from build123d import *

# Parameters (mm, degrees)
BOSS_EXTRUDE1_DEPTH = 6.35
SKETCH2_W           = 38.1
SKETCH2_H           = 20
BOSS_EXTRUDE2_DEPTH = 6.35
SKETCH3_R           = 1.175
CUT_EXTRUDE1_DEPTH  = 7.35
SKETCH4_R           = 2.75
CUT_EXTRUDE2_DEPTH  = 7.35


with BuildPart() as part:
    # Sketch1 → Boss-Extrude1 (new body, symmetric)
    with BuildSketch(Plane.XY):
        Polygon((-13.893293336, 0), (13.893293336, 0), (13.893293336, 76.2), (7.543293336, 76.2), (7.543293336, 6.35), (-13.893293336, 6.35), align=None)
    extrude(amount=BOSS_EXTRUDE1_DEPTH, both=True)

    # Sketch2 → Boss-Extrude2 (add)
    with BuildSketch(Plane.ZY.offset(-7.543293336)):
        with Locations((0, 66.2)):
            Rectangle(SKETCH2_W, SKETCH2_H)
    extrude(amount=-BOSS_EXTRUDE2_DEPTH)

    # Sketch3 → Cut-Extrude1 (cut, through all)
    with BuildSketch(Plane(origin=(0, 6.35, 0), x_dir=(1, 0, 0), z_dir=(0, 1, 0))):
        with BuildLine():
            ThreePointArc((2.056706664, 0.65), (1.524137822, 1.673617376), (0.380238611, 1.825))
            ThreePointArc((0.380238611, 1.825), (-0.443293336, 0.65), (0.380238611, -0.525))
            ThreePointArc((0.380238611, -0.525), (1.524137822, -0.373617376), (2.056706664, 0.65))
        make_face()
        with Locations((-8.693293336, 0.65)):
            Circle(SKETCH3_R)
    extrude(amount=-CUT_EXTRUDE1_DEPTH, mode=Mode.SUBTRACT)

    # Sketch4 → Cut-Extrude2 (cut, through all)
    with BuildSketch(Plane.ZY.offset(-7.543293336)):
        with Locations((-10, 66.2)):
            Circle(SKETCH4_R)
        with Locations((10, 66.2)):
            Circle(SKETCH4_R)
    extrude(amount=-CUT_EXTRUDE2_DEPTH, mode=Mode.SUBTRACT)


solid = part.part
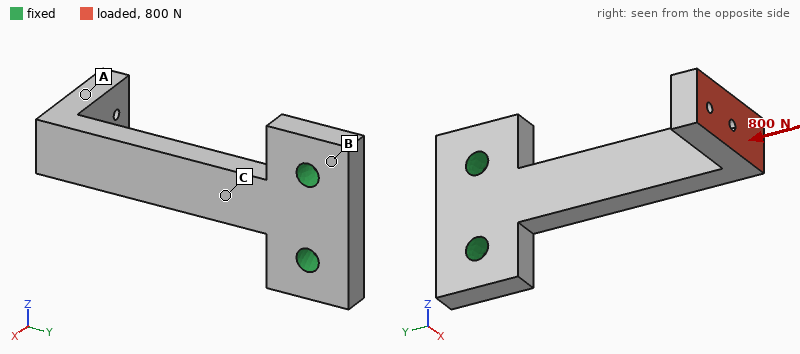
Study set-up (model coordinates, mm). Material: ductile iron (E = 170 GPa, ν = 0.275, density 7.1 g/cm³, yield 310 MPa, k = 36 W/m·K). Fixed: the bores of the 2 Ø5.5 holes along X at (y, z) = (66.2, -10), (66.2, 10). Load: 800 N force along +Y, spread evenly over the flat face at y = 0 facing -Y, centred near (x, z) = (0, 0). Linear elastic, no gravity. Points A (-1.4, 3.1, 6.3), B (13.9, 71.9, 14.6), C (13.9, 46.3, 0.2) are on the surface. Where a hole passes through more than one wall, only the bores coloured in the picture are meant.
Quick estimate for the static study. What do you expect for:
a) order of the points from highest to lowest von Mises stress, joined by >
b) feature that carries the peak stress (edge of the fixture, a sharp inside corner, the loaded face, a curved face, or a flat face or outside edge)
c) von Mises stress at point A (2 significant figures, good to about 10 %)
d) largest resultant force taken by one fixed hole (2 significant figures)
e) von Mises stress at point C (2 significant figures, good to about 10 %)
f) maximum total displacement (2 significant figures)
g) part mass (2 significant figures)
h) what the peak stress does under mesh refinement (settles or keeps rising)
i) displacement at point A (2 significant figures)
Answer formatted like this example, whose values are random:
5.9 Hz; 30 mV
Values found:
C > A > B; a sharp inside corner; 17 MPa; 420 N; 89 MPa; 0.47 mm; 76 g; keeps rising; 0.36 mm
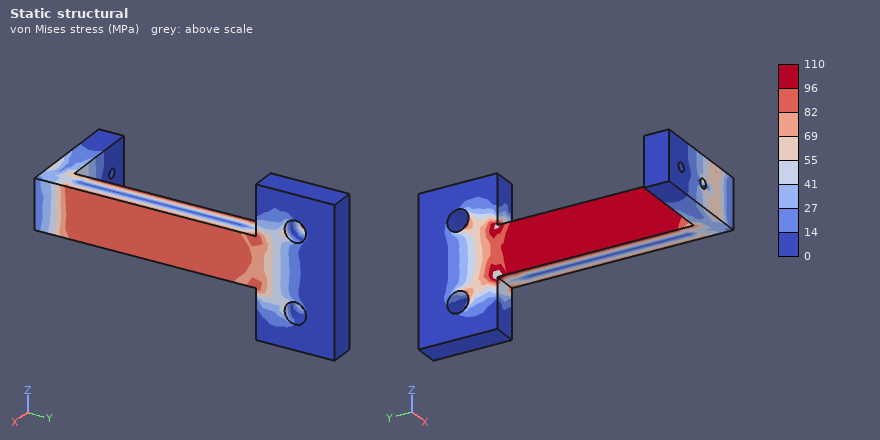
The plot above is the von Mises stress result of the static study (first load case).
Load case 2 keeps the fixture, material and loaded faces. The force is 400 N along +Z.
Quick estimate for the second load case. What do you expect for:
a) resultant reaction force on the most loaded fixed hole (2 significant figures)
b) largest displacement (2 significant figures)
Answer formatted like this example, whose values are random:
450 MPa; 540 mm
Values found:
1.4 kN; 0.28 mm
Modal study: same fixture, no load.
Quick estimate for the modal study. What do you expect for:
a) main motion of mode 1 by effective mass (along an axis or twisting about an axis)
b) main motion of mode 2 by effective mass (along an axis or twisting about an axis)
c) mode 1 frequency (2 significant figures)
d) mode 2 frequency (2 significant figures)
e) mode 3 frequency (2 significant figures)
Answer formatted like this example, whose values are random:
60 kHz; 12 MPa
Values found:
along X; along Z; 830 Hz; 1700 Hz; 3800 Hz
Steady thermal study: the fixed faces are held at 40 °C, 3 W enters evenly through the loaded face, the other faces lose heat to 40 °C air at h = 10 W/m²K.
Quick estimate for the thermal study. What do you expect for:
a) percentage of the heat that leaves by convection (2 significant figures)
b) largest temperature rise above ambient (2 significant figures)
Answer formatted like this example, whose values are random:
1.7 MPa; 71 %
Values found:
30 %; 55 K
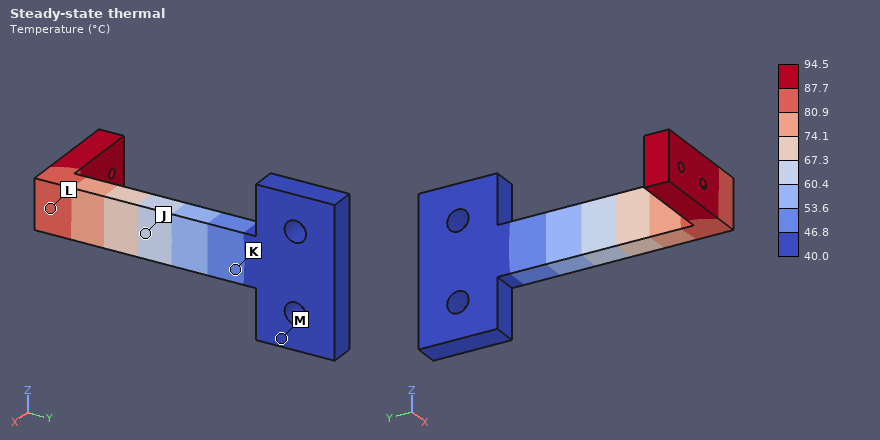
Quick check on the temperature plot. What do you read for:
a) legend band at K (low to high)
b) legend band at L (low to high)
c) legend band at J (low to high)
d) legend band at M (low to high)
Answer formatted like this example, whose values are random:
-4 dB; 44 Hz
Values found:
46.8 to 53.6 °C; 80.9 to 87.7 °C; 60.4 to 67.3 °C; 40.0 to 46.8 °C
